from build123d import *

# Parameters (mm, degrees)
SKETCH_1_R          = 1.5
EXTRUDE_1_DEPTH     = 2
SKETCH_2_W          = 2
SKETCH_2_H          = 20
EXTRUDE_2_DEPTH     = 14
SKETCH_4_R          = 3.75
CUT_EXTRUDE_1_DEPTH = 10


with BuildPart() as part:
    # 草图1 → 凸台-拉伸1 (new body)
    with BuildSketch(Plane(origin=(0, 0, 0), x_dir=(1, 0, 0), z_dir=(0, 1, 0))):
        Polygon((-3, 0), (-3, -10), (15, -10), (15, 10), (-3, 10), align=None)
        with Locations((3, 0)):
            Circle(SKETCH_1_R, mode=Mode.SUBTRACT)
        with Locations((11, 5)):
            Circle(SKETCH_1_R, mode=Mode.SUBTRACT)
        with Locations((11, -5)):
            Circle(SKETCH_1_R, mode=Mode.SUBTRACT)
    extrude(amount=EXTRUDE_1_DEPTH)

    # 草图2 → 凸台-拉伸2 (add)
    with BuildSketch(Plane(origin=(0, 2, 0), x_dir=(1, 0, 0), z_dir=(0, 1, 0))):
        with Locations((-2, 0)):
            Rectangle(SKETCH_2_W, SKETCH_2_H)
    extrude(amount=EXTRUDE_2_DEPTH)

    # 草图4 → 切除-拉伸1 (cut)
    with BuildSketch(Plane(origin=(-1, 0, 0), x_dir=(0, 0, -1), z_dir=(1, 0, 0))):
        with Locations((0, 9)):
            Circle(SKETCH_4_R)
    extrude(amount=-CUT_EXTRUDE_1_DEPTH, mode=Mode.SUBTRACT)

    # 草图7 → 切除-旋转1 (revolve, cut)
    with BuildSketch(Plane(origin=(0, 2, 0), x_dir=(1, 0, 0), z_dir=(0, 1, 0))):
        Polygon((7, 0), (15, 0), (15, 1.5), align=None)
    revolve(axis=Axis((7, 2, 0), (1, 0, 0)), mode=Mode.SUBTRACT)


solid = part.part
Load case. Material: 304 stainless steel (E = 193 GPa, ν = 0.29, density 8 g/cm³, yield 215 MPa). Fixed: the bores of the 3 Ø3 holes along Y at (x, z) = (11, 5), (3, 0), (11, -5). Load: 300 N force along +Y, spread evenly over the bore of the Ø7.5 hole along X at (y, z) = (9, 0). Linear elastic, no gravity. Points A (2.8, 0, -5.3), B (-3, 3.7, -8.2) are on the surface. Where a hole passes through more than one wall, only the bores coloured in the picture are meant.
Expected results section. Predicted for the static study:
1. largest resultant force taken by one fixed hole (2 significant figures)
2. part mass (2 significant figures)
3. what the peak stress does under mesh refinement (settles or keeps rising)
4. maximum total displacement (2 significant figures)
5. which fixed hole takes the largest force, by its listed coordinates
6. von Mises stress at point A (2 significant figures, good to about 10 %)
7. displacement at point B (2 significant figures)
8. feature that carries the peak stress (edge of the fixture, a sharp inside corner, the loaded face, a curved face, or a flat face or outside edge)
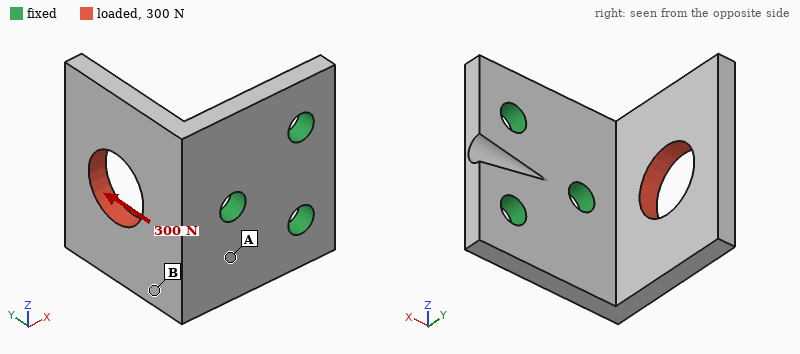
350 N
9.1 g
keeps rising
24 µm
(3, 0)
36 MPa
8.9 µm
edge of the fixture
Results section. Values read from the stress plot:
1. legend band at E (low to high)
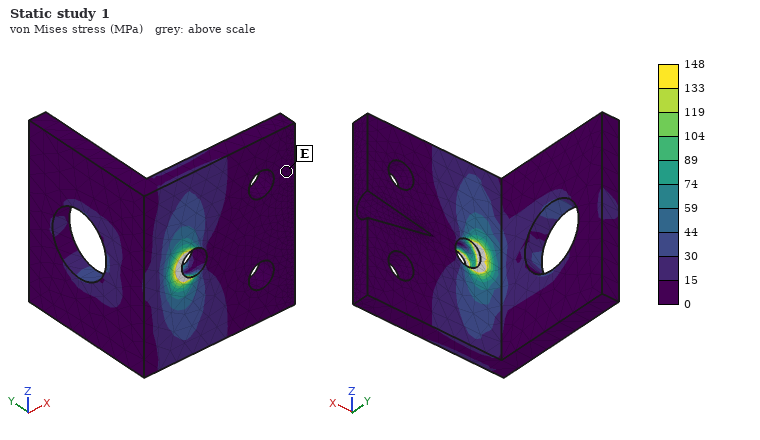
0 to 15 MPa
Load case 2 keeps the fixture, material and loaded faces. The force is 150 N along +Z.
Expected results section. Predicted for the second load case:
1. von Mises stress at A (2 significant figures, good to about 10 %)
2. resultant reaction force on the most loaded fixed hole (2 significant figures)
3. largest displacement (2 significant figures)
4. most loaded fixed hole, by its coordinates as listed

32 MPa
160 N
23 µm
(3, 0)
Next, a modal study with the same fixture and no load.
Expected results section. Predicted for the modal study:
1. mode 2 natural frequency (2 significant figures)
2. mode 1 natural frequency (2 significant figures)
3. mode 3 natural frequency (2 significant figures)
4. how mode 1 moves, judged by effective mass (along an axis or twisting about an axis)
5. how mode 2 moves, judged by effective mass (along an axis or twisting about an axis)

6900 Hz
4900 Hz
11 kHz
along X
along Z
